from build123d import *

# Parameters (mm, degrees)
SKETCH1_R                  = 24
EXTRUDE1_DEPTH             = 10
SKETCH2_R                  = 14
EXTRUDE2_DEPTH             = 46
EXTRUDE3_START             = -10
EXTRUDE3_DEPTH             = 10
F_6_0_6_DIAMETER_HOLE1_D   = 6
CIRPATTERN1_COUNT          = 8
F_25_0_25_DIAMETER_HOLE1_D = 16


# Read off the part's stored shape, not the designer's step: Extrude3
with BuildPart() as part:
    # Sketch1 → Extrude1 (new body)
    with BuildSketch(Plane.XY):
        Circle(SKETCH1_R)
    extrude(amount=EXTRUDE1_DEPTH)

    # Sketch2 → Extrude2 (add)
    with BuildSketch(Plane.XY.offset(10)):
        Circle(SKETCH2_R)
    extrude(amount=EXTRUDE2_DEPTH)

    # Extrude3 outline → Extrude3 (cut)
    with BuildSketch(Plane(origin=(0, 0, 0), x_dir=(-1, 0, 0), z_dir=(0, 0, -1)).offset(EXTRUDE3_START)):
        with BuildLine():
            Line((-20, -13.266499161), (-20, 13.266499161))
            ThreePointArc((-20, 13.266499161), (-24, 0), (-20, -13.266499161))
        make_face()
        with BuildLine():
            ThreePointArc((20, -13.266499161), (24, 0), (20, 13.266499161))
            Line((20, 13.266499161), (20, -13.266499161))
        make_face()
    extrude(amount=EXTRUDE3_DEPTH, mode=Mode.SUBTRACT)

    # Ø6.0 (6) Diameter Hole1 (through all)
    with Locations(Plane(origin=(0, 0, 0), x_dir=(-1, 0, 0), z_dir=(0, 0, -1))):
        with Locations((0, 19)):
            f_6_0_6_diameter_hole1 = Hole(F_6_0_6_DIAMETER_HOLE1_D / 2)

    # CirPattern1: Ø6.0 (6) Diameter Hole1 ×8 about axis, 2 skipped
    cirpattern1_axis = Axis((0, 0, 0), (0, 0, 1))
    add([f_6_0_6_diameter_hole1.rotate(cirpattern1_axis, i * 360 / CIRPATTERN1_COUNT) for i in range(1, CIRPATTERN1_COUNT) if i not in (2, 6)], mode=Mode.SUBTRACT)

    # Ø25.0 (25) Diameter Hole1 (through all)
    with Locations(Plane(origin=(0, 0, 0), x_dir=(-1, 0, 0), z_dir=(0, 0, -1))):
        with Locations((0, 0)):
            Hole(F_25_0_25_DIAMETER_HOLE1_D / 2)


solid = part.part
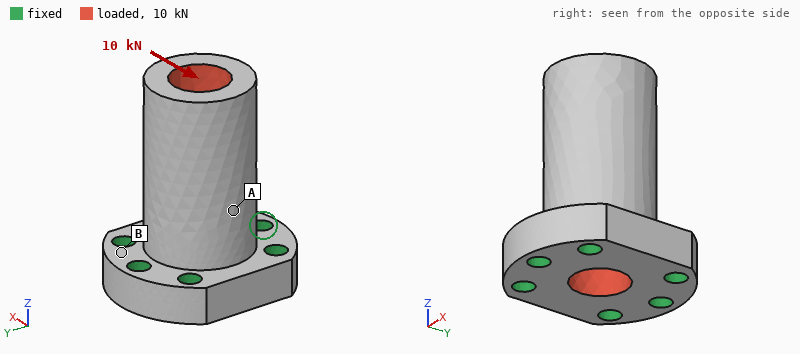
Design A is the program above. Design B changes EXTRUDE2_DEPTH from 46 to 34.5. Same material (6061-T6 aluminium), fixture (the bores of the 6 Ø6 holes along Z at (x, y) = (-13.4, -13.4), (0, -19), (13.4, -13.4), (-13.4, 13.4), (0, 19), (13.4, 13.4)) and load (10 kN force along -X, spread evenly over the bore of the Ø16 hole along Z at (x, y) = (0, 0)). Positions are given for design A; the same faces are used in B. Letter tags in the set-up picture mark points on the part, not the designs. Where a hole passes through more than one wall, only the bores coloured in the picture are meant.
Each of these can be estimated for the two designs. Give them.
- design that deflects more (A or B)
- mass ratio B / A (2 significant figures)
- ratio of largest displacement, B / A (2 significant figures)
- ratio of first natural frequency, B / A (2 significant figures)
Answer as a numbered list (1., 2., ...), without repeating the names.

1. A
2. 0.85
3. 0.54
4. 1.5
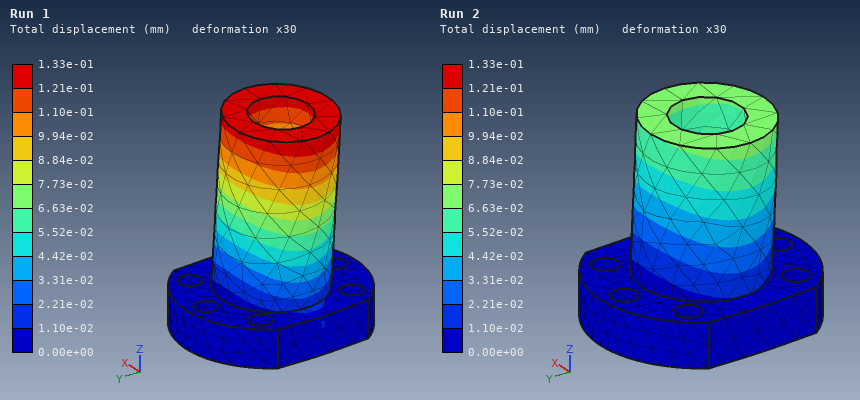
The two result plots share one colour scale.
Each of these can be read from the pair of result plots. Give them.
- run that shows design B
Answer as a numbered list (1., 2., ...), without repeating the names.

1. Run 2
